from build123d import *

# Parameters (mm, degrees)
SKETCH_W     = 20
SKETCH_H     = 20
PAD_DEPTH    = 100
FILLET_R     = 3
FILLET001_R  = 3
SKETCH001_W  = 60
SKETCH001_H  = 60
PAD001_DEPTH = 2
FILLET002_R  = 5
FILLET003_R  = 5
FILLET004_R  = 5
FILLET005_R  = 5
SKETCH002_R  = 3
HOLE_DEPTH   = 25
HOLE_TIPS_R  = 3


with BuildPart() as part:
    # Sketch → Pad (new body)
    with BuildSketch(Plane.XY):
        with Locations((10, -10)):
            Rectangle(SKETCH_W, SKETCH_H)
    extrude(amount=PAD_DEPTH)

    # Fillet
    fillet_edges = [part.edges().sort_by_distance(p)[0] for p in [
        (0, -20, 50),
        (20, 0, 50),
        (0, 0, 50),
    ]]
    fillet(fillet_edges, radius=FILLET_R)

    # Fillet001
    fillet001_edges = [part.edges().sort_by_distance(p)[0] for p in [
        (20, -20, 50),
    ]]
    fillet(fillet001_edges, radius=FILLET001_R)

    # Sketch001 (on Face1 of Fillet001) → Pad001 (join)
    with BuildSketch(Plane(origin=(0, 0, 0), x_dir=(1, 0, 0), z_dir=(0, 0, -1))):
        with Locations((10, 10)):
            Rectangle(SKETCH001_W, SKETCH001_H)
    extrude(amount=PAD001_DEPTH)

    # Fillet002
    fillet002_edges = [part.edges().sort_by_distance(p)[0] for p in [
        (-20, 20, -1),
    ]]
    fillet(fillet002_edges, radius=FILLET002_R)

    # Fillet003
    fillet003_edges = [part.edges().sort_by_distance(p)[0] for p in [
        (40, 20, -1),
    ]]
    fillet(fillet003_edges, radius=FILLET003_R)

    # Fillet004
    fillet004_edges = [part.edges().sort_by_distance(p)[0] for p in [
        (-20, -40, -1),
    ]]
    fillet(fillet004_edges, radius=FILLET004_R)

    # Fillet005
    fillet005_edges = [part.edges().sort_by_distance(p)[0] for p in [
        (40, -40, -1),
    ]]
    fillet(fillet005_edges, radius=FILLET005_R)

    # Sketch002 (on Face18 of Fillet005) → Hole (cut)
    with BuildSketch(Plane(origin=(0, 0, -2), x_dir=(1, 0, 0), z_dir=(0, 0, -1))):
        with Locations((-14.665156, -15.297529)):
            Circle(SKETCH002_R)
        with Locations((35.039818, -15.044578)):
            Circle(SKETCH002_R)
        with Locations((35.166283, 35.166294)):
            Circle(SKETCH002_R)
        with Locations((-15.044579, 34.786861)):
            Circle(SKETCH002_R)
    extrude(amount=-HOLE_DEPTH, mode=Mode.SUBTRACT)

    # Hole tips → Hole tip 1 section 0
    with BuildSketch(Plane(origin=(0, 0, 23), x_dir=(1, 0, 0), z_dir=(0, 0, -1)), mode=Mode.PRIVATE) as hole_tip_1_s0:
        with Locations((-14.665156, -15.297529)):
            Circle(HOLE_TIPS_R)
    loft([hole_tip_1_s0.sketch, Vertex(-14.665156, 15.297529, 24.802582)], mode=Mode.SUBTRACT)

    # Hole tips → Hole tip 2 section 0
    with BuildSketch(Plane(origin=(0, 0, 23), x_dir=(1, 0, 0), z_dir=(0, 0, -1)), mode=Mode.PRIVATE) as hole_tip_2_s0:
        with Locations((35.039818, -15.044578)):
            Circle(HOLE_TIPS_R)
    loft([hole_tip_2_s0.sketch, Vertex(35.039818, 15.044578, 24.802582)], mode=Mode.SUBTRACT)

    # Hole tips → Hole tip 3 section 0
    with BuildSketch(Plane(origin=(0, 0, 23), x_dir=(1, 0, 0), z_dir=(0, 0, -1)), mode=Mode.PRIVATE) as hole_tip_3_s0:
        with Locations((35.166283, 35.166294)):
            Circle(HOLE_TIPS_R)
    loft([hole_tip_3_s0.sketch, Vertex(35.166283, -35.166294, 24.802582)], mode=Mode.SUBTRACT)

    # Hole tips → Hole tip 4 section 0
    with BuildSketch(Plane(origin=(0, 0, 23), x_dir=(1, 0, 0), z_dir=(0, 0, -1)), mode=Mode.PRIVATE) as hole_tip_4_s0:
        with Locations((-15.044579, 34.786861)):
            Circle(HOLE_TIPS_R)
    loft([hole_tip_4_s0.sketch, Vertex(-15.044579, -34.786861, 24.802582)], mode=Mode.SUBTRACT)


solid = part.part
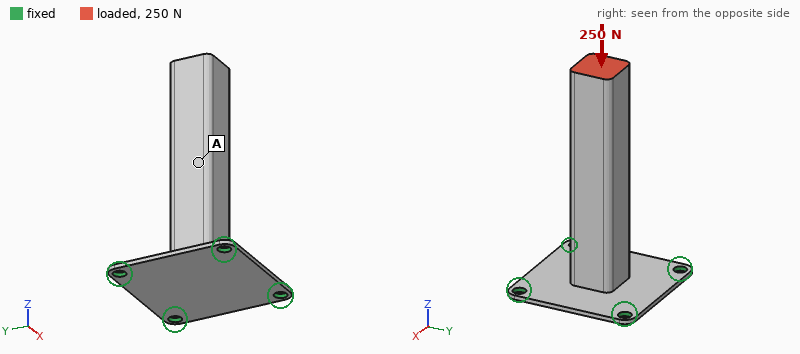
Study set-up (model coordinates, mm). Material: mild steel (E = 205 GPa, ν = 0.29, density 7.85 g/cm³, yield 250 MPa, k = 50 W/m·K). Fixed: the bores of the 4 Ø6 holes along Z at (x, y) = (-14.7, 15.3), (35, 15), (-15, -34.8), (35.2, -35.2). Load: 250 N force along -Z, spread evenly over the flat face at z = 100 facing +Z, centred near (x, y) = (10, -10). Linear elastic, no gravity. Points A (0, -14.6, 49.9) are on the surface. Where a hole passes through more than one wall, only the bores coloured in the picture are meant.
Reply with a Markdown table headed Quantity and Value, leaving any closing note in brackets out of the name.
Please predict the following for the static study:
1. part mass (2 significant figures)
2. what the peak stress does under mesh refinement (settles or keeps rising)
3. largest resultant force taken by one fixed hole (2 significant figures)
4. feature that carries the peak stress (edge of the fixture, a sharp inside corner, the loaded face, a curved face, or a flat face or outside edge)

| Quantity | Value |
|---|---|
| part mass | 360 g |
| what the peak stress does under mesh refinement | keeps rising |
| largest resultant force taken by one fixed hole | 67 N |
| feature that carries the peak stress | edge of the fixture |
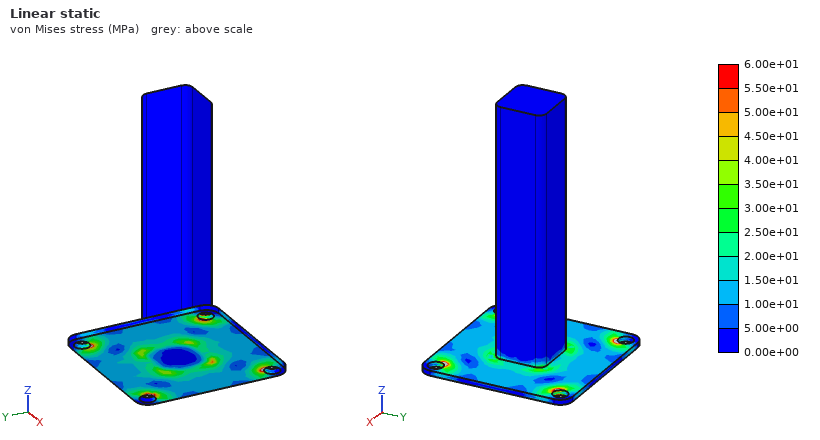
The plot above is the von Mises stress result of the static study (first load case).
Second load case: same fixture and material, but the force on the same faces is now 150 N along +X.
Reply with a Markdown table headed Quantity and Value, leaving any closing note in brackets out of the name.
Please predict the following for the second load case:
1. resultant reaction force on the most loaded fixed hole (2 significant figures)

| Quantity | Value |
|---|---|
| resultant reaction force on the most loaded fixed hole | 200 N |
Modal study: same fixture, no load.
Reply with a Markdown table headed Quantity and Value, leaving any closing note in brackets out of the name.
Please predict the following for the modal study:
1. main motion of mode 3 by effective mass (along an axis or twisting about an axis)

| Quantity | Value |
|---|---|
| main motion of mode 3 by effective mass | along Z |
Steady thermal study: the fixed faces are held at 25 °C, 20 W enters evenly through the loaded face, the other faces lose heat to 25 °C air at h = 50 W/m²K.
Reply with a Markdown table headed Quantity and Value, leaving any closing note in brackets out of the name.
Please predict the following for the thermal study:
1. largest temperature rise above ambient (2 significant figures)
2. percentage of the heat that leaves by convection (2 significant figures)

| Quantity | Value |
|---|---|
| largest temperature rise above ambient | 72 K |
| percentage of the heat that leaves by convection | 80 % |
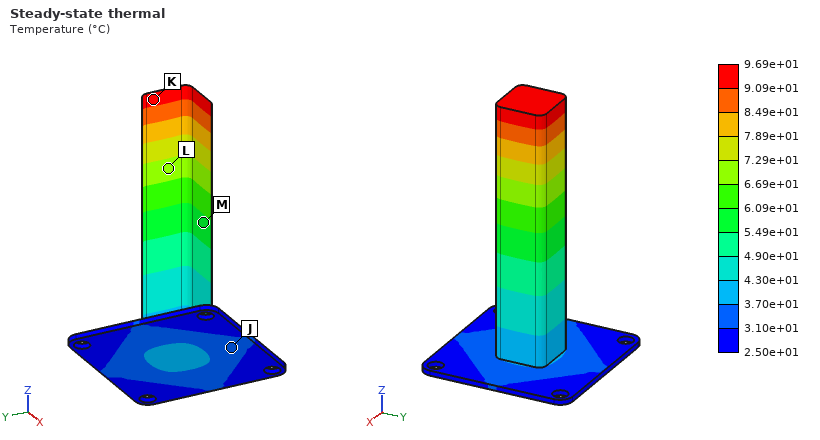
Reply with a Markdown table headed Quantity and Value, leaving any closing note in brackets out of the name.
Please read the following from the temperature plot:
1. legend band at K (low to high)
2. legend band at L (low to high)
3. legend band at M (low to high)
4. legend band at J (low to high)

| Quantity | Value |
|---|---|
| legend band at K | 9.09e+01 to 9.69e+01 °C |
| legend band at L | 6.69e+01 to 7.29e+01 °C |
| legend band at M | 5.49e+01 to 6.09e+01 °C |
| legend band at J | 3.10e+01 to 3.70e+01 °C |
